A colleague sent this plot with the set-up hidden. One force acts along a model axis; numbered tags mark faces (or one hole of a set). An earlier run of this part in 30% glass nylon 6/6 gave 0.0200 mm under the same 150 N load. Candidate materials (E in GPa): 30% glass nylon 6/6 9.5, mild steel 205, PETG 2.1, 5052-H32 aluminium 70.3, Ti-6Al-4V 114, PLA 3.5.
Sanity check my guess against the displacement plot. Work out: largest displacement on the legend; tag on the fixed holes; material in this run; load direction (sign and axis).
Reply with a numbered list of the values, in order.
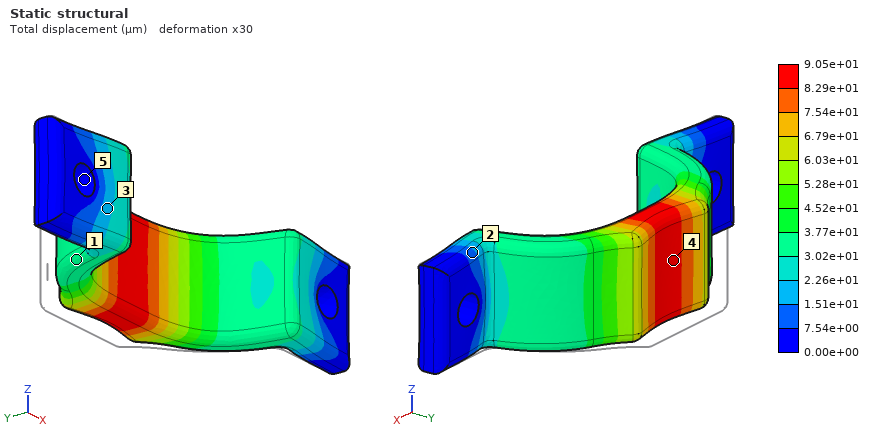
1. 9.05e+01 µm
2. 5
3. PETG
4. -Y
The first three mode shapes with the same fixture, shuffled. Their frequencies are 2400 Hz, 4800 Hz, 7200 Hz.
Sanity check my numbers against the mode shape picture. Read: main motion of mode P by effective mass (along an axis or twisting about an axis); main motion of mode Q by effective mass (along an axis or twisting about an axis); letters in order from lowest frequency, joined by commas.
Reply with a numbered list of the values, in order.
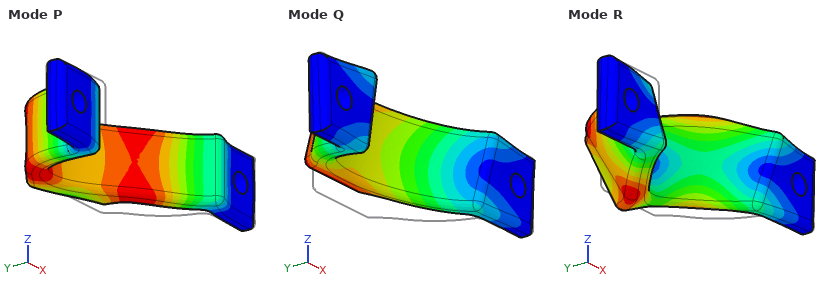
1. along X
2. along Z
3. Q, P, R
